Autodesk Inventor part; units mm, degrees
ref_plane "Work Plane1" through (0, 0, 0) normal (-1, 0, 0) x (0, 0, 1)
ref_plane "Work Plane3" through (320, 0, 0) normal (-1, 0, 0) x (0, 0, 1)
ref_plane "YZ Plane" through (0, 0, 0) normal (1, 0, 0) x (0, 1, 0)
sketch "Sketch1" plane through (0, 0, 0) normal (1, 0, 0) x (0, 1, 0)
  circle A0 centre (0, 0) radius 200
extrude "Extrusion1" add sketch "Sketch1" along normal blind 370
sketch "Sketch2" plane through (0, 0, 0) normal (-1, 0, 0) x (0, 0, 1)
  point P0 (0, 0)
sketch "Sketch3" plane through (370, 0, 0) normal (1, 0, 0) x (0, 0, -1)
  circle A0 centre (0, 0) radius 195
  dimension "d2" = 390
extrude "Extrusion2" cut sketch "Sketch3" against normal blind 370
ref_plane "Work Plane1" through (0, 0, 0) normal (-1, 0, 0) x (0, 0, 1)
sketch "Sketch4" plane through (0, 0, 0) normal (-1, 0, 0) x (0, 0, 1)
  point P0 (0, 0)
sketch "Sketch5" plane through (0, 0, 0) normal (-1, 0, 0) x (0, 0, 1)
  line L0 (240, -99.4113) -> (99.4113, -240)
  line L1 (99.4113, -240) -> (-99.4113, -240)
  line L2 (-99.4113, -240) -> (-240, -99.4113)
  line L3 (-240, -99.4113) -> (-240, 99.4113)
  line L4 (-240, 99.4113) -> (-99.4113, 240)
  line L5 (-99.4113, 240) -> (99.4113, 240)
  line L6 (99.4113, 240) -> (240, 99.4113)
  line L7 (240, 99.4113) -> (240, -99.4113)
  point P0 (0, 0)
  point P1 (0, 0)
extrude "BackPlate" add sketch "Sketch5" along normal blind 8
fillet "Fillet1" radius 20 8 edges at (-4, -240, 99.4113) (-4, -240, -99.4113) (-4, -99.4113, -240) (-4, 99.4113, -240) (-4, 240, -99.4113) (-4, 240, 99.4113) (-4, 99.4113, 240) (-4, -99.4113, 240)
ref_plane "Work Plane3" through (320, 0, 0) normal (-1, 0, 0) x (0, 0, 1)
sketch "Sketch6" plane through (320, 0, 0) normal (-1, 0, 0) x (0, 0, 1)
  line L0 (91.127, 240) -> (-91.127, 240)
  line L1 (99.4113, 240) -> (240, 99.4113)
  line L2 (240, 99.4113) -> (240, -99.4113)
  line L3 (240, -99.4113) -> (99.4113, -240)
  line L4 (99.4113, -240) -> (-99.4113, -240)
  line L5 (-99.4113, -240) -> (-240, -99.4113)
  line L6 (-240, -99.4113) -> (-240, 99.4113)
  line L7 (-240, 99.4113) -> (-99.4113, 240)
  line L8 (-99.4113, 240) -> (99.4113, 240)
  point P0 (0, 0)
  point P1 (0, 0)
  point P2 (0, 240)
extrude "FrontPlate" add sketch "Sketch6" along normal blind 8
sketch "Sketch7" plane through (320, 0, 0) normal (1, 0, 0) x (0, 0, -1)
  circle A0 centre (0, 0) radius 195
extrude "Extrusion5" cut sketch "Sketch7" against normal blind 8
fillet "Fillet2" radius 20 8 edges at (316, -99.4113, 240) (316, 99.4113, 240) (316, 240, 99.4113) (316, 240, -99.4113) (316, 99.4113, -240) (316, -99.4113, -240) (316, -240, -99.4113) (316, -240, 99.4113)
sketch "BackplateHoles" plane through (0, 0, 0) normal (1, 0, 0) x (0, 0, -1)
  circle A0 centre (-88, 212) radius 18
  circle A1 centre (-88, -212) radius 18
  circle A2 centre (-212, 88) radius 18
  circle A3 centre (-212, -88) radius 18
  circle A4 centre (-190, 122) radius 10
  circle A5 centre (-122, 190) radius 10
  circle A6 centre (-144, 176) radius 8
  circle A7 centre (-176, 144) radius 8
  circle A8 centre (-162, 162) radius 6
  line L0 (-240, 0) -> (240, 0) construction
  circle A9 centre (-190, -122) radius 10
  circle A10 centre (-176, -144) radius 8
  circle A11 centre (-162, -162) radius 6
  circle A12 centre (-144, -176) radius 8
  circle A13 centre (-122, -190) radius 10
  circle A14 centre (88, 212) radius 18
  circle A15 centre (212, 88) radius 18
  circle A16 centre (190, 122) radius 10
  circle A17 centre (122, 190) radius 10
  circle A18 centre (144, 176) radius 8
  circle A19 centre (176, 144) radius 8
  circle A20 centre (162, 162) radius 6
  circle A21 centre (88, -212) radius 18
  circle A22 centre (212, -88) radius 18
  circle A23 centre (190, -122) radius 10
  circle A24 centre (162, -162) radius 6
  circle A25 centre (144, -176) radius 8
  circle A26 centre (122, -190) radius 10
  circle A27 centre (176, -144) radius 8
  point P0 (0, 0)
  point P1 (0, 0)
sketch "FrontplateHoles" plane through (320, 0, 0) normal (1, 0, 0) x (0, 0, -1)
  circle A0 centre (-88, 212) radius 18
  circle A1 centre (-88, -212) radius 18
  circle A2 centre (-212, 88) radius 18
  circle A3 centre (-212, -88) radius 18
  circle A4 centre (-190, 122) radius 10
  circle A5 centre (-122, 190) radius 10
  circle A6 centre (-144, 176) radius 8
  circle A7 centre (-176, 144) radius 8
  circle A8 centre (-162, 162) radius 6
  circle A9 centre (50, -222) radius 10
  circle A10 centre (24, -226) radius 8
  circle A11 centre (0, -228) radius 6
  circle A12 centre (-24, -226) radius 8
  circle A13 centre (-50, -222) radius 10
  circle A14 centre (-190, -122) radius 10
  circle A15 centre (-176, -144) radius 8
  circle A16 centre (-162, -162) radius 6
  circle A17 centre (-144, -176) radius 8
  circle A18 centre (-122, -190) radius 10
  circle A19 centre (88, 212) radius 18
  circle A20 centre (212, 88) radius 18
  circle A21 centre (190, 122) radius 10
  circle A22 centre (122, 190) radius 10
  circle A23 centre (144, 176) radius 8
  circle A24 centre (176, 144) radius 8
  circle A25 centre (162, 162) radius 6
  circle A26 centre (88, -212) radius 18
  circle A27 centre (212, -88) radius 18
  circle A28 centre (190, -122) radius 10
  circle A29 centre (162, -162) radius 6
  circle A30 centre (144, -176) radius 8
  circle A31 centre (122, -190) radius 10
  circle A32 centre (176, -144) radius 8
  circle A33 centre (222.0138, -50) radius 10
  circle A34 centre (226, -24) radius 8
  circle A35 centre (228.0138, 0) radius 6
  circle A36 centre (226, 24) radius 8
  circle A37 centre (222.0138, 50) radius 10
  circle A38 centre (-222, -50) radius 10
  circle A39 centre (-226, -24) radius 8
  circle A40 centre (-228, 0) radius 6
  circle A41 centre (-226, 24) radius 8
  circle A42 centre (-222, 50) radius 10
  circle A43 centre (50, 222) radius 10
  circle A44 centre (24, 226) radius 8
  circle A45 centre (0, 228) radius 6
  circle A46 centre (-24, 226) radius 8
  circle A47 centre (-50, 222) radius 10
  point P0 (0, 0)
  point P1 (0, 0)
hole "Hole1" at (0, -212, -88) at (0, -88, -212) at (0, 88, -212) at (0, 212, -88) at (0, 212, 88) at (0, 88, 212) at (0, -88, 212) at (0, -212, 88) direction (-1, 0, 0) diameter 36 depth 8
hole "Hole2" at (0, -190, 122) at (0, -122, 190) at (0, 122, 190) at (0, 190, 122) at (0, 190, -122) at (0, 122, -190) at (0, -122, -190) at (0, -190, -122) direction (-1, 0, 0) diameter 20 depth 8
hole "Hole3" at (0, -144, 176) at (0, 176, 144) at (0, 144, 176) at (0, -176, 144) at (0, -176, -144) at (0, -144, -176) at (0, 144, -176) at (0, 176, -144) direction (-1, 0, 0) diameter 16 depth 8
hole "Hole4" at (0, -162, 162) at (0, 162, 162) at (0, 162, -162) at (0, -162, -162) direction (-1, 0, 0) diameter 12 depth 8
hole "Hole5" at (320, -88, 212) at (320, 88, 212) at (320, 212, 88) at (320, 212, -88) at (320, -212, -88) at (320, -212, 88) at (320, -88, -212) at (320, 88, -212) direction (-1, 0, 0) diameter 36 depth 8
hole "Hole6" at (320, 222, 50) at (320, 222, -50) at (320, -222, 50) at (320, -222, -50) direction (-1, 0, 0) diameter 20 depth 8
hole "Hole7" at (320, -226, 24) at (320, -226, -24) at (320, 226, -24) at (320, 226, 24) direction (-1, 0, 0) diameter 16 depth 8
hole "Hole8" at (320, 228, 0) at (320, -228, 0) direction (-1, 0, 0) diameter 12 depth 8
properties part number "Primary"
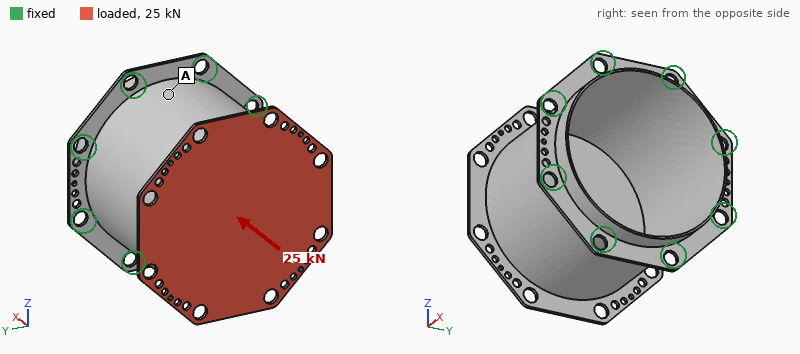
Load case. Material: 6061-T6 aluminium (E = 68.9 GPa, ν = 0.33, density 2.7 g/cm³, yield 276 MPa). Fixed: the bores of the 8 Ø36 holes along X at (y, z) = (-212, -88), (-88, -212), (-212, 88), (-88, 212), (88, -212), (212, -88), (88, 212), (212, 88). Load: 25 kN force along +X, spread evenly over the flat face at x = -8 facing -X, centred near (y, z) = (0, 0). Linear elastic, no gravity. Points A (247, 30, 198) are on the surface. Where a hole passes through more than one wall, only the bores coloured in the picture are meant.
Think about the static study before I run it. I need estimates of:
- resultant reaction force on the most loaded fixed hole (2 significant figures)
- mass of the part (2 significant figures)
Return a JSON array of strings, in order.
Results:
["3.2 kN", "11 kg"]
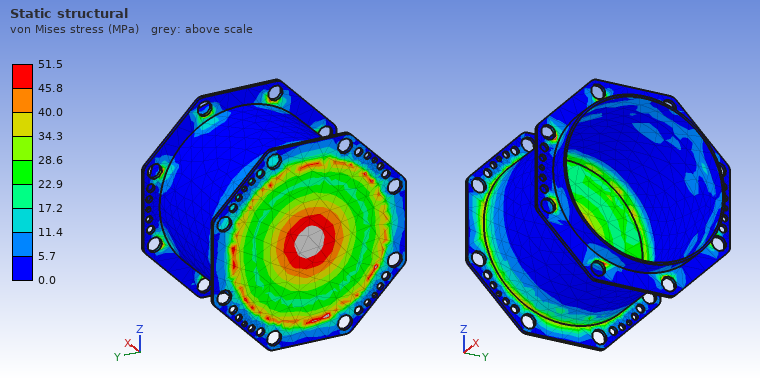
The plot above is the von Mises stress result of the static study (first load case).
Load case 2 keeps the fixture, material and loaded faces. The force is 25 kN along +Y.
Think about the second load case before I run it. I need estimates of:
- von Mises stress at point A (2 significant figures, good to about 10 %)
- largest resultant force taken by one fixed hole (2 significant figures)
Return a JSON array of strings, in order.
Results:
["15 MPa", "9.4 kN"]
